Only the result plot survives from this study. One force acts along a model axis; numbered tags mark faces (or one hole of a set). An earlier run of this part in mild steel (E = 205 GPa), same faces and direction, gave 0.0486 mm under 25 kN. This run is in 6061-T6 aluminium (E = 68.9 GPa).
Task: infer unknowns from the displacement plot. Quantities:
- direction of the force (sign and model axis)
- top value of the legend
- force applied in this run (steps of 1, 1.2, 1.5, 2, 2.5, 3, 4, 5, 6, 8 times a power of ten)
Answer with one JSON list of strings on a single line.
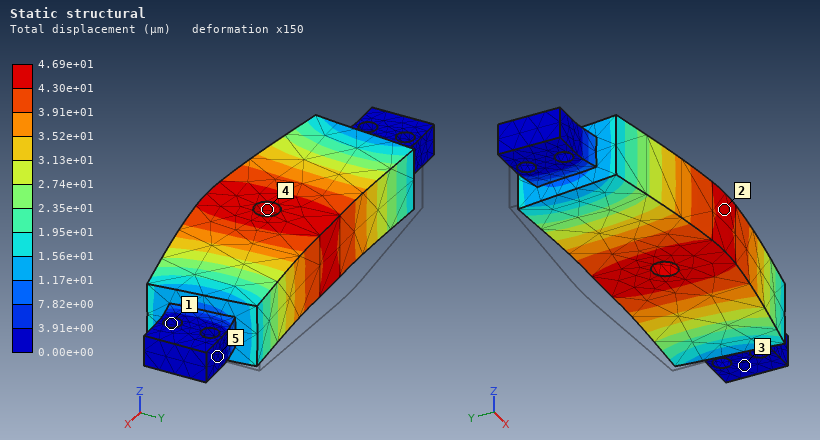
["-Y", "4.69e+01 µm", "8 kN"]
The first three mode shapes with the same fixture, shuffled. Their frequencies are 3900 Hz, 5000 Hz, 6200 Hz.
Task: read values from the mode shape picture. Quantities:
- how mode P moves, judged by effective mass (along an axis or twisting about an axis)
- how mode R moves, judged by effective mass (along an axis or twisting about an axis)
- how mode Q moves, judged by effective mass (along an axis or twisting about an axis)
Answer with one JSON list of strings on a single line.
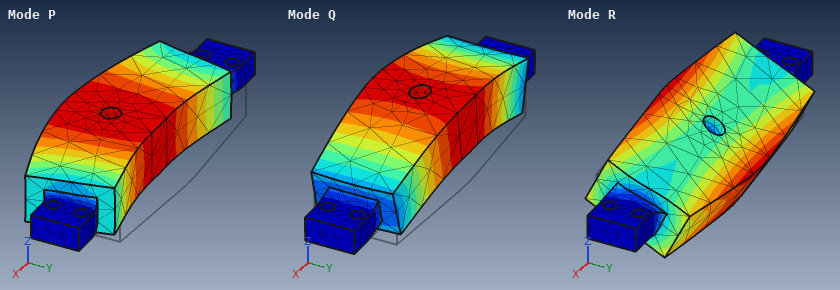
["along Y", "twisting about X", "along Z"]
